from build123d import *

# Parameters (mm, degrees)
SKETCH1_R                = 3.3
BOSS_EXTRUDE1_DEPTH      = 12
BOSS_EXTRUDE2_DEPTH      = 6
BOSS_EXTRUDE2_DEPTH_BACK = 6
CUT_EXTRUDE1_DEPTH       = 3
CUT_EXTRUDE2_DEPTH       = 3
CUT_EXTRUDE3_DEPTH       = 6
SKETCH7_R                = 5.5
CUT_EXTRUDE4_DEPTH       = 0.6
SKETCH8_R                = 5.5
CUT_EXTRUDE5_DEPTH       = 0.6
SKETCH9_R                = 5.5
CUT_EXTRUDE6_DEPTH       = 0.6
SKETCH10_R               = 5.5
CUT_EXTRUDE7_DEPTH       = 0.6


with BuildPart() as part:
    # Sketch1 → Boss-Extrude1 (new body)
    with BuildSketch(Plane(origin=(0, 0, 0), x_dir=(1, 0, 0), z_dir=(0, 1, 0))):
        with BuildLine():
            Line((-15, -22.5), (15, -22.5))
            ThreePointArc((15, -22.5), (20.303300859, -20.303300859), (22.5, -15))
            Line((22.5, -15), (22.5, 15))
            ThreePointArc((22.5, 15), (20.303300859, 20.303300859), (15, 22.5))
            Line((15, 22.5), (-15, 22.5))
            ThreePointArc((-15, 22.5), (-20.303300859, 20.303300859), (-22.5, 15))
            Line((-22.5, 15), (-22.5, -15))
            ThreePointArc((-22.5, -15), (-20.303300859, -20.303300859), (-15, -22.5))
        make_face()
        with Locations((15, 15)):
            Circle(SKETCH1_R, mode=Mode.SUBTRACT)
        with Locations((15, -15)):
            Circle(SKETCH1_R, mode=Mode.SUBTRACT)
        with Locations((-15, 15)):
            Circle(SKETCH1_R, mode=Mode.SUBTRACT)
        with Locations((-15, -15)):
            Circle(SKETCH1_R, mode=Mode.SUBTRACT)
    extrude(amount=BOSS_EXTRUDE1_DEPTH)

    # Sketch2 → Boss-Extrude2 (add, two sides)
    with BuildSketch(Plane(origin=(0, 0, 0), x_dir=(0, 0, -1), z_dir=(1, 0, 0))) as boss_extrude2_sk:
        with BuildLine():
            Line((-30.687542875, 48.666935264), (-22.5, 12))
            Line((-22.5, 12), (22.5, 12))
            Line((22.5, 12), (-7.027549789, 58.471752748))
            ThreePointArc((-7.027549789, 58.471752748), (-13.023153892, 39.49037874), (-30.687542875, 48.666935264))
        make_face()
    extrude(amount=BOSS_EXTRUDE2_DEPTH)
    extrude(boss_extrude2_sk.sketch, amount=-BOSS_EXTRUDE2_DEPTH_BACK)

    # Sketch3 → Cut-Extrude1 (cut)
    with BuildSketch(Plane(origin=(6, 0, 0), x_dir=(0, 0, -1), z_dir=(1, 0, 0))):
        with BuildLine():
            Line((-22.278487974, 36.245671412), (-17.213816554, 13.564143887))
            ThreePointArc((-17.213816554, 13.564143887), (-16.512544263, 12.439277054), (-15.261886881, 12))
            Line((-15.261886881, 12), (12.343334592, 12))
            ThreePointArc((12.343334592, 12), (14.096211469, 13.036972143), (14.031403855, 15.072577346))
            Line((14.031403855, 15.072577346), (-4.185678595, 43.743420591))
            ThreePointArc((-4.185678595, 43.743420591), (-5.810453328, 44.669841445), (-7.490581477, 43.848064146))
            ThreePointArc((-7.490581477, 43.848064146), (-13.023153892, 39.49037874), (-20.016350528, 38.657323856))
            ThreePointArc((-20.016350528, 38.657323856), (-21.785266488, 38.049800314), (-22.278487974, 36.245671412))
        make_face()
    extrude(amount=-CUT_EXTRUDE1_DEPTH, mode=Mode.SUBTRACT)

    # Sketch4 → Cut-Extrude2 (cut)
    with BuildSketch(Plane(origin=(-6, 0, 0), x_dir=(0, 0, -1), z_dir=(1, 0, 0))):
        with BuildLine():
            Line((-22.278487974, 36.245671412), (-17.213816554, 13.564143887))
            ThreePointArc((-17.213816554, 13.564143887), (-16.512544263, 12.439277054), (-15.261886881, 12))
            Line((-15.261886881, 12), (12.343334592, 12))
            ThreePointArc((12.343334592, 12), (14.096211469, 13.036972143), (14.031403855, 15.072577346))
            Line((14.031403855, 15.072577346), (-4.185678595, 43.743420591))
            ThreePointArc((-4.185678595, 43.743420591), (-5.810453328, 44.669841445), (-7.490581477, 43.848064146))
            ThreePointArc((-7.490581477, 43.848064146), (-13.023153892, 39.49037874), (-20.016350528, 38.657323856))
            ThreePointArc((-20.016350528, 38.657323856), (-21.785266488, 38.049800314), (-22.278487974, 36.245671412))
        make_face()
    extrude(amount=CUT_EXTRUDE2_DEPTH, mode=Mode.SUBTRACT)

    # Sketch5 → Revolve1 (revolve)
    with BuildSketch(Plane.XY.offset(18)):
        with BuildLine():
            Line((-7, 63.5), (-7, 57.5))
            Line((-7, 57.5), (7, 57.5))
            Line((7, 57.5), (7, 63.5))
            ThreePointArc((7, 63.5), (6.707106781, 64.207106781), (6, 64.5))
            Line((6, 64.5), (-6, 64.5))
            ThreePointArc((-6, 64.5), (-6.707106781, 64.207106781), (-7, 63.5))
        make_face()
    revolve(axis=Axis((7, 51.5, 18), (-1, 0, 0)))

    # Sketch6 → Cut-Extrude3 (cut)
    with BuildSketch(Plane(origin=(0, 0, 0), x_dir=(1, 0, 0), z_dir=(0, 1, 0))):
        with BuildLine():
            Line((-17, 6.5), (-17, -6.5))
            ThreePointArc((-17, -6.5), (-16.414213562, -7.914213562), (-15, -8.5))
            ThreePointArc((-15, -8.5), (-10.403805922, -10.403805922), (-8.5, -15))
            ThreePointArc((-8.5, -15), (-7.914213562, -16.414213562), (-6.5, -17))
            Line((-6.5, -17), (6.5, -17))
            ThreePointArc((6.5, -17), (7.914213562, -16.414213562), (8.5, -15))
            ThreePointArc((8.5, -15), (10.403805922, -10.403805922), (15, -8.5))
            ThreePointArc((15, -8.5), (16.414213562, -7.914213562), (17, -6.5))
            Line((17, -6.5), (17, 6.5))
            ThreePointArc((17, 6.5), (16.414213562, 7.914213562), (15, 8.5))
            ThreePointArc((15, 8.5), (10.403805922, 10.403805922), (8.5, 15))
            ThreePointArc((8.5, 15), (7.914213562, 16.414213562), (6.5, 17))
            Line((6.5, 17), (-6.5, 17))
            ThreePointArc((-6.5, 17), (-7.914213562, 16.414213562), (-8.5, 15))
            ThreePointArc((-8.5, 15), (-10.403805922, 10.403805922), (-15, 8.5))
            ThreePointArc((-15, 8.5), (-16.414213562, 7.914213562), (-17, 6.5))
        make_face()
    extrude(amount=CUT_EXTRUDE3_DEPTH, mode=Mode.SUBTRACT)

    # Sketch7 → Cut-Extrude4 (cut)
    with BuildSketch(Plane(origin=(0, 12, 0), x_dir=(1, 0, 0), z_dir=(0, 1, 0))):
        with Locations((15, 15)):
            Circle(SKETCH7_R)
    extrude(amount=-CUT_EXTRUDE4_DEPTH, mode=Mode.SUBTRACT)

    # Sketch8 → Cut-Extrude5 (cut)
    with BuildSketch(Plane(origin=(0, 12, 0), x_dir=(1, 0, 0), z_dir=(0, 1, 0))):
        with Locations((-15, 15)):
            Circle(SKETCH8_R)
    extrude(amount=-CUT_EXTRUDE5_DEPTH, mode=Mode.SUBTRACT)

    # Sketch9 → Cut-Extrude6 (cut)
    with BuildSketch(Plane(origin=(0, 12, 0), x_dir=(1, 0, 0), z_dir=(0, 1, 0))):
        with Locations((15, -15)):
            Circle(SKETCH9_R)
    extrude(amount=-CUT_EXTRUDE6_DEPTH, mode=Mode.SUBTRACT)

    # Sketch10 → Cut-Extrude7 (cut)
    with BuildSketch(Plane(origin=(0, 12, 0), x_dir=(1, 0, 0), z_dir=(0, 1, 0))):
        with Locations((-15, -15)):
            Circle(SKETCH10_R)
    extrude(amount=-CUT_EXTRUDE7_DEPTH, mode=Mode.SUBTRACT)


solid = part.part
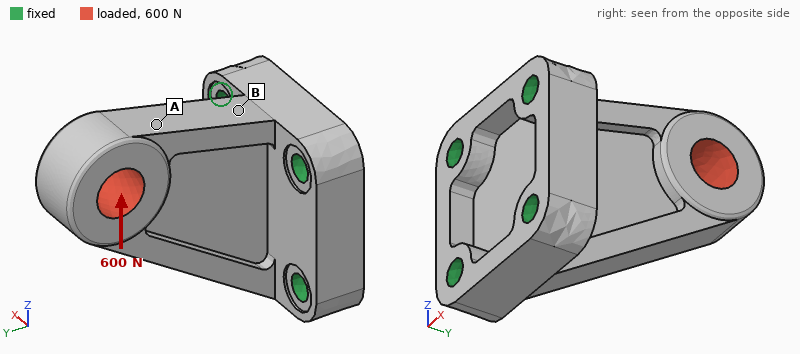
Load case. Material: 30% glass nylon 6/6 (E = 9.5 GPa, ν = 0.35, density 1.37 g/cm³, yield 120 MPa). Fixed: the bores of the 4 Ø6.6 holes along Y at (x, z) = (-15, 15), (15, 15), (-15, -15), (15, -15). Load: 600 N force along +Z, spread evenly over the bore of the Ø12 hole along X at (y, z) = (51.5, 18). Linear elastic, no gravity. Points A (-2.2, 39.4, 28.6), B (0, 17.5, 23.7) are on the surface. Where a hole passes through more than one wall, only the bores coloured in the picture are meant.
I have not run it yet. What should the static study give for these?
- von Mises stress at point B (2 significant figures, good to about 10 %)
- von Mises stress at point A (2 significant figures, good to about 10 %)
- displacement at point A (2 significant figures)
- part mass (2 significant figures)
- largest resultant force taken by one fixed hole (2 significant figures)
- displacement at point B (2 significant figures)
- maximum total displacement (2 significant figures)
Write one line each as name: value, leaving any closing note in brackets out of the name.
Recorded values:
von Mises stress at point B: 7.6 MPa
von Mises stress at point A: 3.0 MPa
displacement at point A: 0.083 mm
part mass: 44 g
largest resultant force taken by one fixed hole: 440 N
displacement at point B: 0.033 mm
maximum total displacement: 0.13 mm
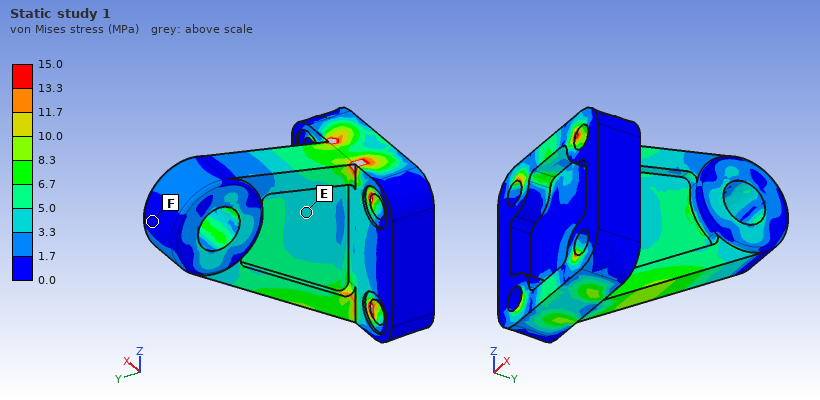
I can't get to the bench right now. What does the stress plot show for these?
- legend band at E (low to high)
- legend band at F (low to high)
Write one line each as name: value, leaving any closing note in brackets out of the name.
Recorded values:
legend band at E: 3.3 to 5.0 MPa
legend band at F: 0.0 to 1.7 MPa
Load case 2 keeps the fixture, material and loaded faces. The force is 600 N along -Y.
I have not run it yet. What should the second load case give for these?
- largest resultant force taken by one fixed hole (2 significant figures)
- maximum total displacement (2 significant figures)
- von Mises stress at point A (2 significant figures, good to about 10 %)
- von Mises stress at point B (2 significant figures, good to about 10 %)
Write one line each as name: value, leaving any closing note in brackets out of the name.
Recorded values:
largest resultant force taken by one fixed hole: 320 N
maximum total displacement: 51 µm
von Mises stress at point A: 3.5 MPa
von Mises stress at point B: 5.5 MPa
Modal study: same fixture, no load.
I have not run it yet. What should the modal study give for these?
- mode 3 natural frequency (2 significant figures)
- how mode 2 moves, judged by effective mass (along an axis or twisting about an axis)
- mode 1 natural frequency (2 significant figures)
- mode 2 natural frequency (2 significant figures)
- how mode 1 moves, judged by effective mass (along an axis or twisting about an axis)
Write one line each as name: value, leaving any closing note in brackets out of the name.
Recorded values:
mode 3 natural frequency: 4100 Hz
how mode 2 moves, judged by effective mass: along Z
mode 1 natural frequency: 1300 Hz
mode 2 natural frequency: 3500 Hz
how mode 1 moves, judged by effective mass: along X
